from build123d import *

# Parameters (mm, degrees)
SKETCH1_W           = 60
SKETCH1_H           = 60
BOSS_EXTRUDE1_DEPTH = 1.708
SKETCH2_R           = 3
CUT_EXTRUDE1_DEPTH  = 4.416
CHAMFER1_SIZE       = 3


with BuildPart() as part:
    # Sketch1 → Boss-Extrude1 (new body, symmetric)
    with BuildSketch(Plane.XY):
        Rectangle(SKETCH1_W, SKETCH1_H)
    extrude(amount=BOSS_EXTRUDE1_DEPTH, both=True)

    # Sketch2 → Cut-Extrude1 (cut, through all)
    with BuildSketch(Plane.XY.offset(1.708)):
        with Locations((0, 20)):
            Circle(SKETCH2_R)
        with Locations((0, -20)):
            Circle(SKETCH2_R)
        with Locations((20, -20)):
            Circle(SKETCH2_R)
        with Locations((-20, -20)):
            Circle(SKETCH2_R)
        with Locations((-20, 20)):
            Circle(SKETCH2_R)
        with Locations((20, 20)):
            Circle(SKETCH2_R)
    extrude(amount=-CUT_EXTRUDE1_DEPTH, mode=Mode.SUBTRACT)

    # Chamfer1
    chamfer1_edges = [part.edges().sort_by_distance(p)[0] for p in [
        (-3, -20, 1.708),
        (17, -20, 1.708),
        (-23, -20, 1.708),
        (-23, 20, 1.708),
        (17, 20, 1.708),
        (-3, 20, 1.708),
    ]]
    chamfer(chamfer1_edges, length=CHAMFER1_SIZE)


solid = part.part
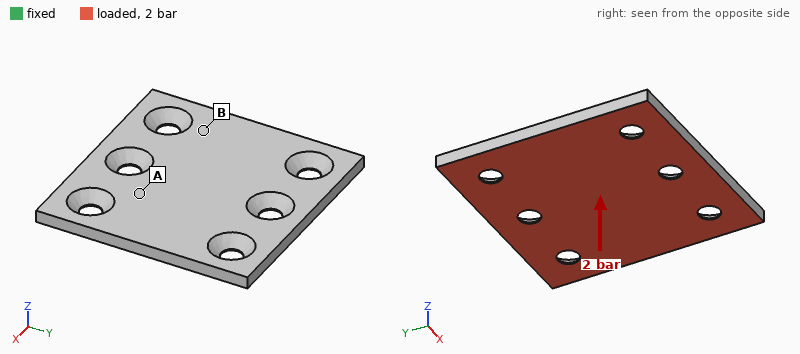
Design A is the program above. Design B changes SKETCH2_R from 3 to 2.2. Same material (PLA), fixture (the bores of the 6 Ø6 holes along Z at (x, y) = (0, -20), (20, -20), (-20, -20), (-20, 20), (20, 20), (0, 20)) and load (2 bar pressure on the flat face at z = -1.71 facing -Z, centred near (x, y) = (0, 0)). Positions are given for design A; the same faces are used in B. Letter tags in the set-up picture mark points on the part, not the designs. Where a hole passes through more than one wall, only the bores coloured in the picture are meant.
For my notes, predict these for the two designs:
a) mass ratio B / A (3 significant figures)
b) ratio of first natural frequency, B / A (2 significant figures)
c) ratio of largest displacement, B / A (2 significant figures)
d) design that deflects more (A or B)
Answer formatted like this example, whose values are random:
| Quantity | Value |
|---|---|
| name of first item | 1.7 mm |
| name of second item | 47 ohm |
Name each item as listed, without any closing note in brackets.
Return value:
| Quantity | Value |
|---|---|
| mass ratio B / A | 1.04 |
| ratio of first natural frequency, B / A | 0.88 |
| ratio of largest displacement, B / A | 1.2 |
| design that deflects more | B |
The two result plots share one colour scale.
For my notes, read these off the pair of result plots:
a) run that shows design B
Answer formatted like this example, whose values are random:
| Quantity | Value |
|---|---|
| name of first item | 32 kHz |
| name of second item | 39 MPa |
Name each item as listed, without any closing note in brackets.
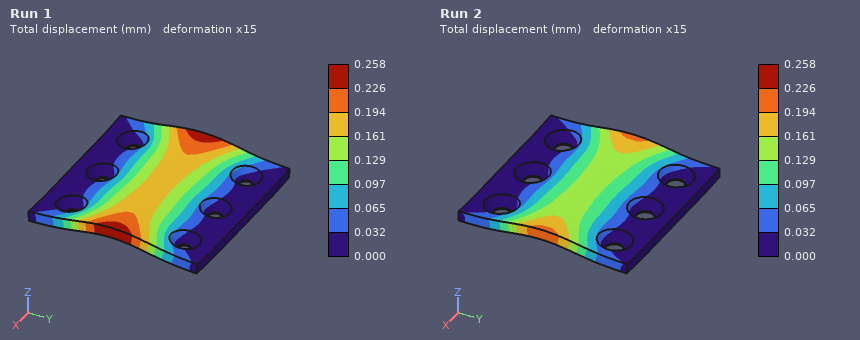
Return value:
| Quantity | Value |
|---|---|
| run that shows design B | Run 1 |
